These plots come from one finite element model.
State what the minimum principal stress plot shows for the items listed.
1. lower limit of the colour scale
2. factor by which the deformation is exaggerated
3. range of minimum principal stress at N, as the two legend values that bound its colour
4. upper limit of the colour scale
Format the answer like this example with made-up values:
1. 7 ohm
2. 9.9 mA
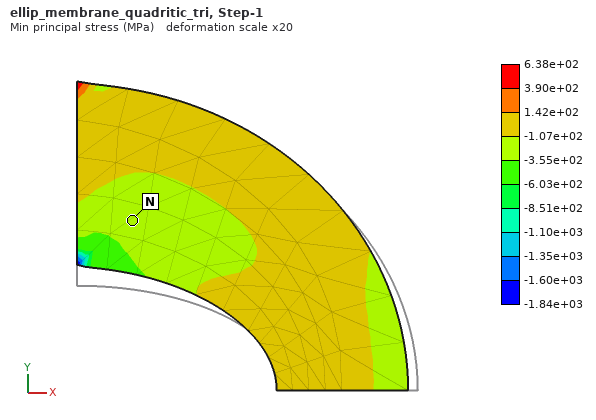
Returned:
1. -1.84e+03 MPa
2. 20
3. -3.55e+02 to -1.07e+02 MPa
4. 6.38e+02 MPa
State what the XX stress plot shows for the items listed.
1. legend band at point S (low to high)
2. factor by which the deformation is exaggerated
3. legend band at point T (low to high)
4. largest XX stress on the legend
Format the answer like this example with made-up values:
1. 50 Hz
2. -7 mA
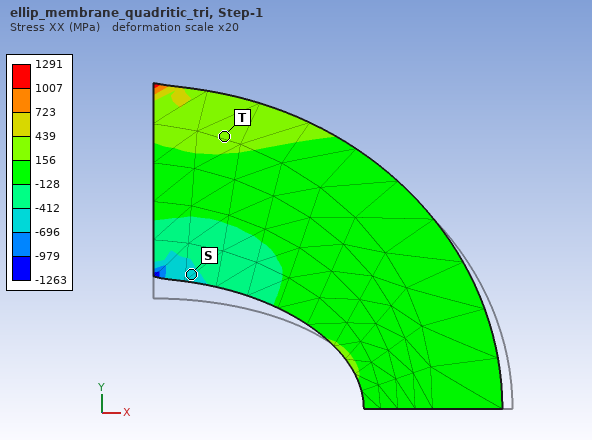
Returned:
1. -696 to -412 MPa
2. 20
3. 156 to 439 MPa
4. 1291 MPa
